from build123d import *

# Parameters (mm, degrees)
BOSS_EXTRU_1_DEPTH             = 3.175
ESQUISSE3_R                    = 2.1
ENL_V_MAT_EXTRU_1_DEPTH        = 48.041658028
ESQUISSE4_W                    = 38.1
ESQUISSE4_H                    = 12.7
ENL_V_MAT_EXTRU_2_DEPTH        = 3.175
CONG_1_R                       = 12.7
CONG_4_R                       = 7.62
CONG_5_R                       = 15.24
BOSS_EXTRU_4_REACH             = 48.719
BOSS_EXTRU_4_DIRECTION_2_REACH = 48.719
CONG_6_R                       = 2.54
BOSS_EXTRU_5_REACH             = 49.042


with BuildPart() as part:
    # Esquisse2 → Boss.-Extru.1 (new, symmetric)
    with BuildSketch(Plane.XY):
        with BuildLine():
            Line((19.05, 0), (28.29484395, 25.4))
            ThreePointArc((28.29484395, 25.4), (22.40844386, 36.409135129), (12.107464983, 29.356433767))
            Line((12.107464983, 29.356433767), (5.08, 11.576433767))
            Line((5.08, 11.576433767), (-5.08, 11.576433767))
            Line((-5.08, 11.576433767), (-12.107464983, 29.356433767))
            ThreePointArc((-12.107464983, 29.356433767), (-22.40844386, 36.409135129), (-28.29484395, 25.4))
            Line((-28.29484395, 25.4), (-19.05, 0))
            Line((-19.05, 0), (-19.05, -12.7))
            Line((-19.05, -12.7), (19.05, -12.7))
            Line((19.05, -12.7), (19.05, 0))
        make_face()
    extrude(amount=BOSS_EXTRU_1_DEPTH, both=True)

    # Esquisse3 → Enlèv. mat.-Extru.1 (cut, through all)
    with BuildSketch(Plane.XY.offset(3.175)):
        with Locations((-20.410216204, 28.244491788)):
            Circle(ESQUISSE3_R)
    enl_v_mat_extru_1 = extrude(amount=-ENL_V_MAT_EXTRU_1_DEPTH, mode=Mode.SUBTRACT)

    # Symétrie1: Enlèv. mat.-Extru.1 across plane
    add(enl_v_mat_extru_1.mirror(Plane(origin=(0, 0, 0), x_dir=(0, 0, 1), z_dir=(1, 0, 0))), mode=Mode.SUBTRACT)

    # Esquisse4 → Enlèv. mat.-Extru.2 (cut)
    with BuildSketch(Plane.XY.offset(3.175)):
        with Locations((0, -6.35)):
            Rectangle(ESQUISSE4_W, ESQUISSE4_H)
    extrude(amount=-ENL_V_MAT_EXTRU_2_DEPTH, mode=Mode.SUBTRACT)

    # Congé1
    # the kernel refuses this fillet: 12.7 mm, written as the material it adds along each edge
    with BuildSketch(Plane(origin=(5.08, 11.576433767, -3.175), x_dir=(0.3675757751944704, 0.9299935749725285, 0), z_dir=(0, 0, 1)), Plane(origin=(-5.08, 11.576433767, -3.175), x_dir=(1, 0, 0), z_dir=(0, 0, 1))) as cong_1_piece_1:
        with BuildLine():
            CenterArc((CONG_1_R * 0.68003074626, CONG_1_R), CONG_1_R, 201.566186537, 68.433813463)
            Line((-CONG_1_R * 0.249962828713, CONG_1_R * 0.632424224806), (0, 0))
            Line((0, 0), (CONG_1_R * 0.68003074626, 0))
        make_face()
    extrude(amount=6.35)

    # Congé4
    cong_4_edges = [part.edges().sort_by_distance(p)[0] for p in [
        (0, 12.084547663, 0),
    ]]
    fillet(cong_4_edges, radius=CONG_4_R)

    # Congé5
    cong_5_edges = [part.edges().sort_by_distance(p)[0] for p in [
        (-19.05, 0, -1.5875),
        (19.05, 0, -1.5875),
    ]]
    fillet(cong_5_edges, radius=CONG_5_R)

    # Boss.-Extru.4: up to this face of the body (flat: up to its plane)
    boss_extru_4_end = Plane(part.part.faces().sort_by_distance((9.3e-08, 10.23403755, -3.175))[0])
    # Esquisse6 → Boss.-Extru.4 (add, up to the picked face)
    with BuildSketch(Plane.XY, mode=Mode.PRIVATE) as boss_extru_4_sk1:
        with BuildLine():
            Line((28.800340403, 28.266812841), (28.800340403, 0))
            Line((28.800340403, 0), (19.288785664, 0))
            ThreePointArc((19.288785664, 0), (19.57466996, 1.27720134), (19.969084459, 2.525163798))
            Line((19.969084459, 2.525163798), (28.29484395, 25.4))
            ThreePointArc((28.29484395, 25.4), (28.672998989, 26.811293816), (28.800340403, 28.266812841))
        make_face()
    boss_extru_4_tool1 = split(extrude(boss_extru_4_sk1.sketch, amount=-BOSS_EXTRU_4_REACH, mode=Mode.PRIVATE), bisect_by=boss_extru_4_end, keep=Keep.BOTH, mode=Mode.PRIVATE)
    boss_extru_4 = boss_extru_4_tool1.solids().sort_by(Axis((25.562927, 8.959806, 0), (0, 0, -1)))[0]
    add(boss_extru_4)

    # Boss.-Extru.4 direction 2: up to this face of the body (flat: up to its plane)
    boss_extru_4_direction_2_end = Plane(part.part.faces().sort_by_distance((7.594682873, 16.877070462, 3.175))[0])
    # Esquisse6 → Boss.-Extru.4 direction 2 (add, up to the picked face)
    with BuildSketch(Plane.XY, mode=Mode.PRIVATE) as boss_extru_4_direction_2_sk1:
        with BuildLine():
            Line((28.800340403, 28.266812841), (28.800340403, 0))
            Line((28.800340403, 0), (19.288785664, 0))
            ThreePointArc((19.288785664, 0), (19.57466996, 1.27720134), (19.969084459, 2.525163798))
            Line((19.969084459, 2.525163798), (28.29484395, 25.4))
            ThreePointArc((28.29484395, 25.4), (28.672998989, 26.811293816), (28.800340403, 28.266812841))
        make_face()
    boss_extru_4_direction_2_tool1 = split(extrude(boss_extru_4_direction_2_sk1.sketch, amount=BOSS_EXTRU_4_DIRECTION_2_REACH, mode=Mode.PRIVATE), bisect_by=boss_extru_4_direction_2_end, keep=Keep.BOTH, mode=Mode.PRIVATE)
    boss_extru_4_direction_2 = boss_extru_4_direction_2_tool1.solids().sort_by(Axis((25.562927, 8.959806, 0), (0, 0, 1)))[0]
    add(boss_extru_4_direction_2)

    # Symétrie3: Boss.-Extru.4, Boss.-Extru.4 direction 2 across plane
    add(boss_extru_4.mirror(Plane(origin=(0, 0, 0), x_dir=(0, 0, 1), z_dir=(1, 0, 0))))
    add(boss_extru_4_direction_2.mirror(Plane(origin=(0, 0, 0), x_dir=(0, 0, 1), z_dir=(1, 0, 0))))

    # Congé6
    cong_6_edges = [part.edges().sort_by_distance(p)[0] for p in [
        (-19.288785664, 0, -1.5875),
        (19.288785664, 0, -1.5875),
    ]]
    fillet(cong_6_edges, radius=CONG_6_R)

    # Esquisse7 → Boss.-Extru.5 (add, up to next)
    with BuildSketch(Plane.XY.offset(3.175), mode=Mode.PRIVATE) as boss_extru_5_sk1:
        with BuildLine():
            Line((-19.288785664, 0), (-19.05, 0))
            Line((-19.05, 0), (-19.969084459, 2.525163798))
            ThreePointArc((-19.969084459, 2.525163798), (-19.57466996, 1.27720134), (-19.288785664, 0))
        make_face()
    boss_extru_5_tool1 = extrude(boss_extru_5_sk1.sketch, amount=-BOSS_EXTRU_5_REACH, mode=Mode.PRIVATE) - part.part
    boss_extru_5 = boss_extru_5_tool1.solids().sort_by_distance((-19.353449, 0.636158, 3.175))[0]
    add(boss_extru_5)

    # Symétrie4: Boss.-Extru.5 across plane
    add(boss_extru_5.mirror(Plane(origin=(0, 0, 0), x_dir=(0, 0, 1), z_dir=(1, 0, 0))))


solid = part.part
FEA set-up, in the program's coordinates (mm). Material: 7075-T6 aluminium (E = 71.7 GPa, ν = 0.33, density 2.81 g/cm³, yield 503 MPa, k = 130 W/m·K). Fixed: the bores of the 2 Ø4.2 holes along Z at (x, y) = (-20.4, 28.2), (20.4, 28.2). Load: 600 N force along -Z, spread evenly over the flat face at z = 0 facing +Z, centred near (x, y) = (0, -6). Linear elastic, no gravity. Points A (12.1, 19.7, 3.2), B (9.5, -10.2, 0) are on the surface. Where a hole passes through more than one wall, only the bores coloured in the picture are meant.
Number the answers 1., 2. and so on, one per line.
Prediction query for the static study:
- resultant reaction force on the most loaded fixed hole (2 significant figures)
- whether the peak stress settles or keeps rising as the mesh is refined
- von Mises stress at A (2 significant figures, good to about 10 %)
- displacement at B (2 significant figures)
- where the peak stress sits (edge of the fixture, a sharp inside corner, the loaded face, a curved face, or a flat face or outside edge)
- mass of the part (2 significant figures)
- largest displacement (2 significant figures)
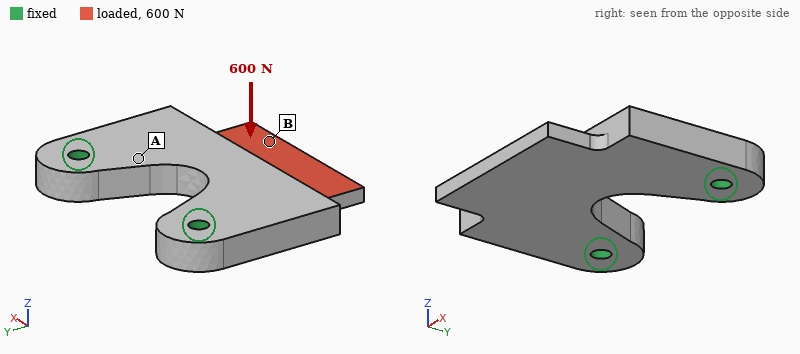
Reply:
1. 300 N
2. keeps rising
3. 54 MPa
4. 0.20 mm
5. edge of the fixture
6. 32 g
7. 0.23 mm
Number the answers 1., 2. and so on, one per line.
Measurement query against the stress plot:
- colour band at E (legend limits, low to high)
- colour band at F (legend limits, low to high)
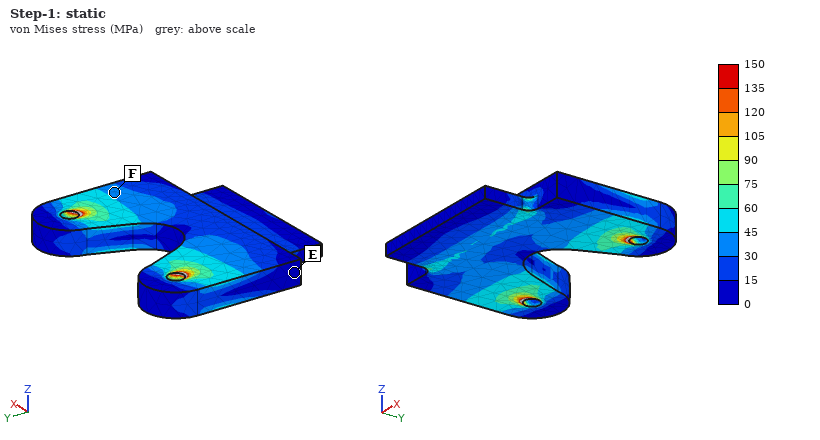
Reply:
1. 0 to 15 MPa
2. 30 to 45 MPa
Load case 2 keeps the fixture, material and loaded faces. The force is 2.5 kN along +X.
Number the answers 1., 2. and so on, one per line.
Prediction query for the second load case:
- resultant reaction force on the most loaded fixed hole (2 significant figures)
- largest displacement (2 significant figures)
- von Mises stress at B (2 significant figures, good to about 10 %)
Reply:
1. 2.2 kN
2. 49 µm
3. 26 MPa
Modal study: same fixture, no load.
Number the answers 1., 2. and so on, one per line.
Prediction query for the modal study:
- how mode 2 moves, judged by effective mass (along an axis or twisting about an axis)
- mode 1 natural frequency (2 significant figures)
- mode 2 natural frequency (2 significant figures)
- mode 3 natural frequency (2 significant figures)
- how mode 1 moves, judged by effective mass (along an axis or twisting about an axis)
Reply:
1. twisting about Y
2. 3400 Hz
3. 7100 Hz
4. 13 kHz
5. along Z
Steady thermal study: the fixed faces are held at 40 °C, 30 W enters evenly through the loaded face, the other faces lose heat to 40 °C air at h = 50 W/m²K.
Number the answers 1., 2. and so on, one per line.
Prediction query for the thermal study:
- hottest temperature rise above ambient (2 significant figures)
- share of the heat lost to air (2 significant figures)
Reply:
1. 38 K
2. 12 %
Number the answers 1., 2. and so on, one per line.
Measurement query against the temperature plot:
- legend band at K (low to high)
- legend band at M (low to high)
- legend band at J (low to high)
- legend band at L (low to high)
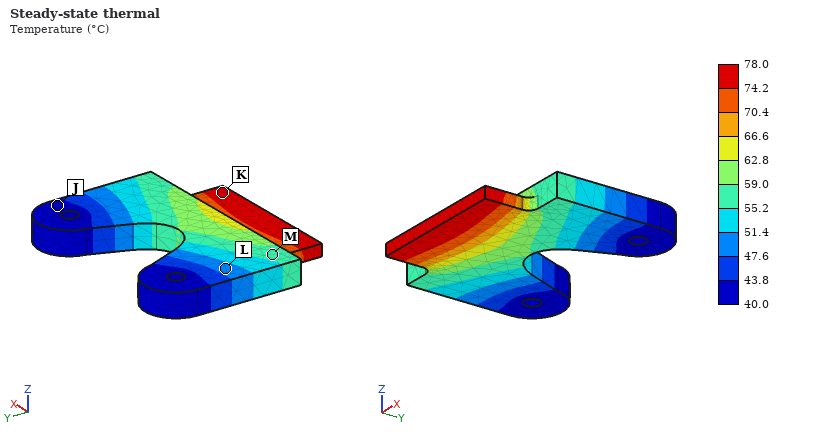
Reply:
1. 74.2 to 78.0 °C
2. 55.2 to 59.0 °C
3. 40.0 to 43.8 °C
4. 47.6 to 51.4 °C
